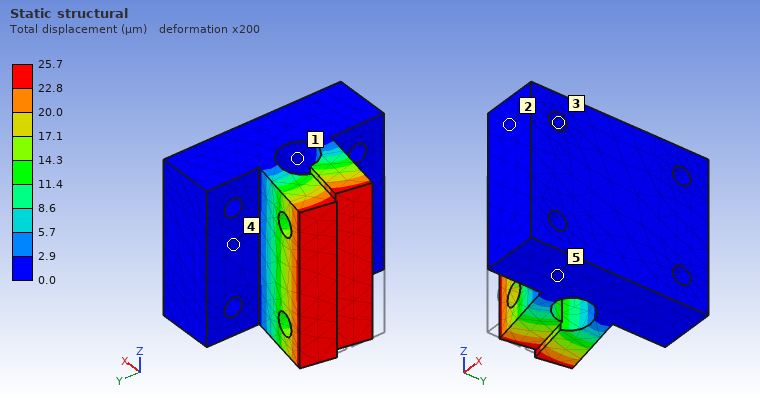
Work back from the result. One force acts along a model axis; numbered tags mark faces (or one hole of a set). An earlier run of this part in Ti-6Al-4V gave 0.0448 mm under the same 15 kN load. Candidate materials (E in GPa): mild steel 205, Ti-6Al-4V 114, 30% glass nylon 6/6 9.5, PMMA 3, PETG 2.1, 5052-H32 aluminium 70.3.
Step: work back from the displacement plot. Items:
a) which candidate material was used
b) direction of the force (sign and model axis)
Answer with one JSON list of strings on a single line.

["mild steel", "+Y"]
